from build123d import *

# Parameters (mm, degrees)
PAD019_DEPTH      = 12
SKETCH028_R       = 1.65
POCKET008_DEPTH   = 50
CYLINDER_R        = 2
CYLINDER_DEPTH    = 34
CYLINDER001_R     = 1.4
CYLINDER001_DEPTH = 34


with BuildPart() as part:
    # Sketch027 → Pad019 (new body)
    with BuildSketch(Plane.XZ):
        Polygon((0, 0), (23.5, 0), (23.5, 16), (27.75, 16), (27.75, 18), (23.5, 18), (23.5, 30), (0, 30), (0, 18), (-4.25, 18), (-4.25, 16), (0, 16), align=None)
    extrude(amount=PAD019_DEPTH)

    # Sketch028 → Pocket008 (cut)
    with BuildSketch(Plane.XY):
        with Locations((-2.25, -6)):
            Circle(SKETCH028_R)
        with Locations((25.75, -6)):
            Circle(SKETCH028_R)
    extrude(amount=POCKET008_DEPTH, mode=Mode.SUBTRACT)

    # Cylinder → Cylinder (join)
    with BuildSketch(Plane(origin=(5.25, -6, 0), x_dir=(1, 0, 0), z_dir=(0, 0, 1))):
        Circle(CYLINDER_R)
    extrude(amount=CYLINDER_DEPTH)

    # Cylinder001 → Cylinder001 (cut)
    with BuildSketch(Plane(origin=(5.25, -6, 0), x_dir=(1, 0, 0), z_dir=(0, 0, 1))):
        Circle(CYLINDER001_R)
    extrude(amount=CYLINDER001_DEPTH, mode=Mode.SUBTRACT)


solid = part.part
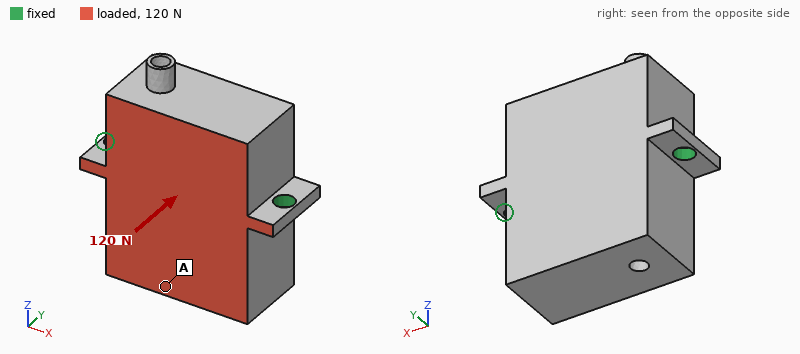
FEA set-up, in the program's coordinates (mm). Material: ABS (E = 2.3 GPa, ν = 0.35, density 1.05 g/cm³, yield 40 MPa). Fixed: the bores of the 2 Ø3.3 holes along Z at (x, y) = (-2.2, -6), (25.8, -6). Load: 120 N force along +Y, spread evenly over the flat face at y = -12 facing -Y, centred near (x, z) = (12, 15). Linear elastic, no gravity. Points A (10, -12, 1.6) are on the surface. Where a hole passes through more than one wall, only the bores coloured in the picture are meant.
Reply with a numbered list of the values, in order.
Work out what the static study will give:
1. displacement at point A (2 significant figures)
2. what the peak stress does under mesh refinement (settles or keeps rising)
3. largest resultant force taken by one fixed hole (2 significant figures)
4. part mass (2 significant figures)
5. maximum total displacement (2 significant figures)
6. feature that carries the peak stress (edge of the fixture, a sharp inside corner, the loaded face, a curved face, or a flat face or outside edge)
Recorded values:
1. 0.12 mm
2. keeps rising
3. 60 N
4. 8.9 g
5. 0.13 mm
6. edge of the fixture
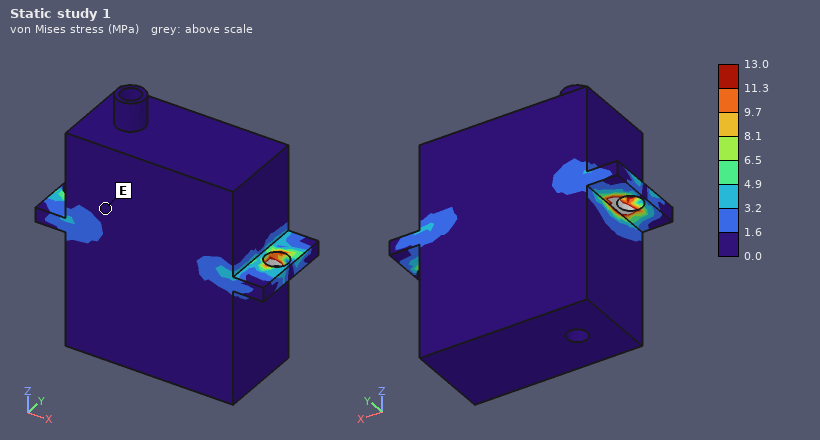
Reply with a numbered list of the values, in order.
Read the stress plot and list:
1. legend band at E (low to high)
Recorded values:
1. 0.0 to 1.6 MPa
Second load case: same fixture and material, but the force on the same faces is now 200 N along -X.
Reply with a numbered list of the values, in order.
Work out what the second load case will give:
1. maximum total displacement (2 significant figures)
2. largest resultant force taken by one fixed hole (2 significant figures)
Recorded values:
1. 31 µm
2. 110 N
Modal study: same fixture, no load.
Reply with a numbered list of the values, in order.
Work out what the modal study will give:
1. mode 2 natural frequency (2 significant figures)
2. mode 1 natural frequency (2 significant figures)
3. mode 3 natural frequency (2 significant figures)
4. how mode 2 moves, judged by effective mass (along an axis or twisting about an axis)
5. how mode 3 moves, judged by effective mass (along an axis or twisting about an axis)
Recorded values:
1. 4600 Hz
2. 1100 Hz
3. 5000 Hz
4. along Y
5. along Z
